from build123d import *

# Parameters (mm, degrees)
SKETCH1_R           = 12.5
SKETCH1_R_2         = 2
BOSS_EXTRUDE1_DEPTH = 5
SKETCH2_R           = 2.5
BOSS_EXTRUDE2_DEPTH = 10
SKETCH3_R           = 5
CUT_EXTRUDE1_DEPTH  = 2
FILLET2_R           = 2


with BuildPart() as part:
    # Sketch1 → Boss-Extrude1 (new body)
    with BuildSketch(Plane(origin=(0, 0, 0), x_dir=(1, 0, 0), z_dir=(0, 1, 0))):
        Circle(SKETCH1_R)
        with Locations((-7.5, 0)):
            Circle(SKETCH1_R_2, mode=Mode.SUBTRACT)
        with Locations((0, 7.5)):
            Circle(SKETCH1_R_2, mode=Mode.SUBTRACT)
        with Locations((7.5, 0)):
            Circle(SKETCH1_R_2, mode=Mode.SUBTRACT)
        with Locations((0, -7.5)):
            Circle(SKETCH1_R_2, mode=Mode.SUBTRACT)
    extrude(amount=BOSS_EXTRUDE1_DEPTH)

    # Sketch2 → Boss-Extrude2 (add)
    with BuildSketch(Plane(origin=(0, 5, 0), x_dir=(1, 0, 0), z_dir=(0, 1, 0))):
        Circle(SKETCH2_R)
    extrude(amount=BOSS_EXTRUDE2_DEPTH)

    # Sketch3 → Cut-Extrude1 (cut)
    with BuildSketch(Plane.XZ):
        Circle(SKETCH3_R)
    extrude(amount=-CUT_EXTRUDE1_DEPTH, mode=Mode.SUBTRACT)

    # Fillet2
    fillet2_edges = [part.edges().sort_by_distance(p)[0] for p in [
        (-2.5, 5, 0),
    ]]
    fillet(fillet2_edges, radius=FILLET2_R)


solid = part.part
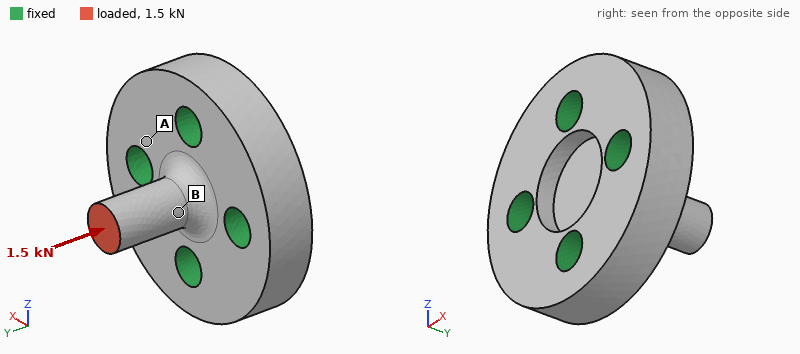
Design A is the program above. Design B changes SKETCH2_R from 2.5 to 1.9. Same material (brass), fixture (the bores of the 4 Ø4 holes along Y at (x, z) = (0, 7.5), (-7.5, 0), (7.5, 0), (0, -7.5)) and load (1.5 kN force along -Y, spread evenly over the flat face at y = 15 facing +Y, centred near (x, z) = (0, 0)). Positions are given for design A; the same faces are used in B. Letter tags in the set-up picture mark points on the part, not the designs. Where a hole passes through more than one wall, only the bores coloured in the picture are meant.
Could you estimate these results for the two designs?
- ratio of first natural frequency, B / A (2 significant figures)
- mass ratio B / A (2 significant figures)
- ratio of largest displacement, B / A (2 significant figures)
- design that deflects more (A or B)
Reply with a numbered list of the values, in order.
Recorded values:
1. 0.85
2. 0.96
3. 1.6
4. B
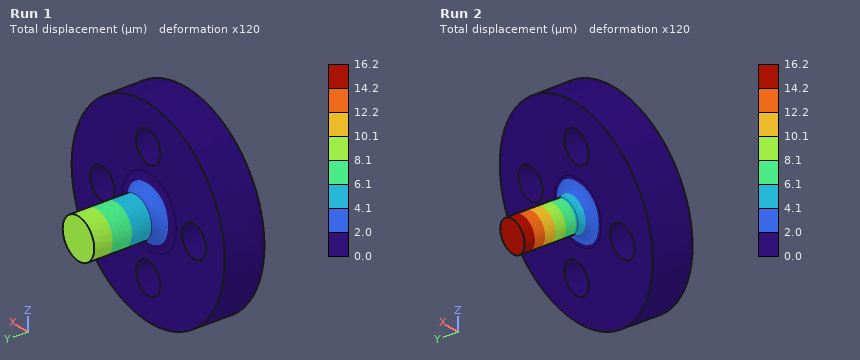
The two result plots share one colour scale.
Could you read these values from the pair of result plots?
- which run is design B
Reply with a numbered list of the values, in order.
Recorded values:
1. Run 2
